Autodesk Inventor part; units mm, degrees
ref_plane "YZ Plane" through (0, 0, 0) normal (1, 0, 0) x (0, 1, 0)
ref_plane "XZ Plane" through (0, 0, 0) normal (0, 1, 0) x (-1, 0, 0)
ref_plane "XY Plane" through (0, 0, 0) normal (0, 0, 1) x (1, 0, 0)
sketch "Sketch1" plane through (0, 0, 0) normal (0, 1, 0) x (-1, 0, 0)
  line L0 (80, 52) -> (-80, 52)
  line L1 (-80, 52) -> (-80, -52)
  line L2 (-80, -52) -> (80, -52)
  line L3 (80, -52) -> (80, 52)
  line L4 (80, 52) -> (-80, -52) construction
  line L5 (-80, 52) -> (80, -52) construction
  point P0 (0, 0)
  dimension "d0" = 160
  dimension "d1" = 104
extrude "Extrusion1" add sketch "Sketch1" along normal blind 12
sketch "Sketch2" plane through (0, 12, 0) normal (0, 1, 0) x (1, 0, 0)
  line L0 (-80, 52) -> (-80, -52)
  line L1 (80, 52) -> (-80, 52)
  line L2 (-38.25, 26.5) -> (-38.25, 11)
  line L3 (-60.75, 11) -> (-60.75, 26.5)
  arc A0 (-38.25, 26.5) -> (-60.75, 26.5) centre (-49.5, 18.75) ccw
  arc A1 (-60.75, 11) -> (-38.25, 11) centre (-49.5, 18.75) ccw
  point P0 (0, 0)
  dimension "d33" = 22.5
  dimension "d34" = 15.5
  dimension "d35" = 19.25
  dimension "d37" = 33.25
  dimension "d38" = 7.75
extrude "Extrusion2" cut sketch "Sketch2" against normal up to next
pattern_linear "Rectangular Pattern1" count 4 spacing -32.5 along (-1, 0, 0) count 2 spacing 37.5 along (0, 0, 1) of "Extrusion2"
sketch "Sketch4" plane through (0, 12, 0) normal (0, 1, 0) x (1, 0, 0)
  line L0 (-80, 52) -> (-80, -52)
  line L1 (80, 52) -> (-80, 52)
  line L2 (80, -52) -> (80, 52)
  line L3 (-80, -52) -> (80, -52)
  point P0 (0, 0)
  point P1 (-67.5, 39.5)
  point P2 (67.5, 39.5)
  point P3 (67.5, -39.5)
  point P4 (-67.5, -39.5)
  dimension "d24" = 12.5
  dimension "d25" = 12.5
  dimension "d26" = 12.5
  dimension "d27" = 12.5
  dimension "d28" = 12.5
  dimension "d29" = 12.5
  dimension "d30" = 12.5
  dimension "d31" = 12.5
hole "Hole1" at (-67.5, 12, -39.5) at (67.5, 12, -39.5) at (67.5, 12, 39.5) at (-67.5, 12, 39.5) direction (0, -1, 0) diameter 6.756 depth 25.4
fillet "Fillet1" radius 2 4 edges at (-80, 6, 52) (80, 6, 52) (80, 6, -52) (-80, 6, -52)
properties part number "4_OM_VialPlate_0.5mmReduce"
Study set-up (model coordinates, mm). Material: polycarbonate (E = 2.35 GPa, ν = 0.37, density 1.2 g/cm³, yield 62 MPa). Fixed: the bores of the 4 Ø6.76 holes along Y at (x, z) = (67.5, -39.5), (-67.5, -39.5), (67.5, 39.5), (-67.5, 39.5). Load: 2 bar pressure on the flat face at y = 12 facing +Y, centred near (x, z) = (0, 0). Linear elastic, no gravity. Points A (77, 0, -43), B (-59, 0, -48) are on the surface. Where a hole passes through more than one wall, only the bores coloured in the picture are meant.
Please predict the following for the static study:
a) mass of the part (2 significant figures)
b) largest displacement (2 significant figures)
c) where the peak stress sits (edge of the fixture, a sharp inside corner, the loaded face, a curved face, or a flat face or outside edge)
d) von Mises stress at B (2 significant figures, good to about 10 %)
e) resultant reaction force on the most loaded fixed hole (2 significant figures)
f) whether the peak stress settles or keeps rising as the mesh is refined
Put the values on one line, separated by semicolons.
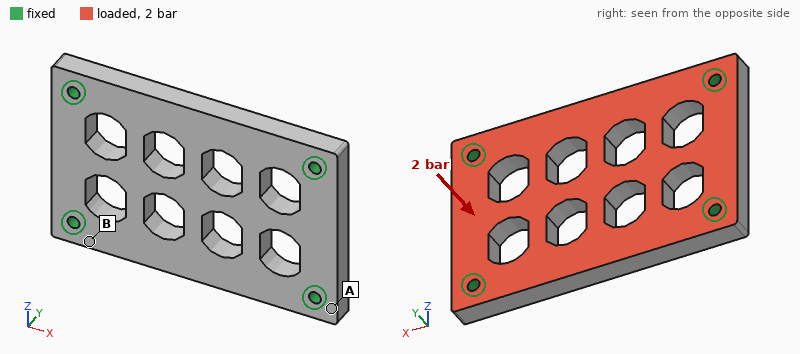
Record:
180 g; 0.83 mm; edge of the fixture; 8.6 MPa; 610 N; keeps rising
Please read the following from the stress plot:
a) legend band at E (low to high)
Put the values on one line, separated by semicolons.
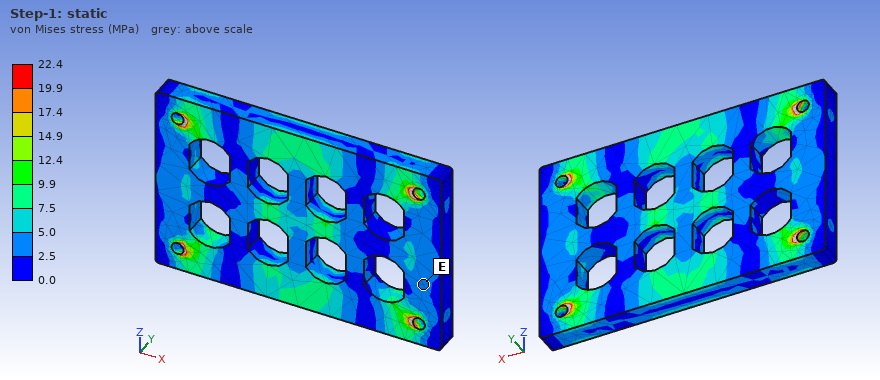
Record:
2.5 to 5.0 MPa
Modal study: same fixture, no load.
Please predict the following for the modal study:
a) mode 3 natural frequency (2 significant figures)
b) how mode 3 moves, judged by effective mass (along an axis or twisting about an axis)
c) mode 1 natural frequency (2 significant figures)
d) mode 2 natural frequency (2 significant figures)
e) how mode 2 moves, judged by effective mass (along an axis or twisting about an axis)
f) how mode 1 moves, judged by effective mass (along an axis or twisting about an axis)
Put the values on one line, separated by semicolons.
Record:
1600 Hz; along Z; 760 Hz; 1000 Hz; twisting about X; along Y
